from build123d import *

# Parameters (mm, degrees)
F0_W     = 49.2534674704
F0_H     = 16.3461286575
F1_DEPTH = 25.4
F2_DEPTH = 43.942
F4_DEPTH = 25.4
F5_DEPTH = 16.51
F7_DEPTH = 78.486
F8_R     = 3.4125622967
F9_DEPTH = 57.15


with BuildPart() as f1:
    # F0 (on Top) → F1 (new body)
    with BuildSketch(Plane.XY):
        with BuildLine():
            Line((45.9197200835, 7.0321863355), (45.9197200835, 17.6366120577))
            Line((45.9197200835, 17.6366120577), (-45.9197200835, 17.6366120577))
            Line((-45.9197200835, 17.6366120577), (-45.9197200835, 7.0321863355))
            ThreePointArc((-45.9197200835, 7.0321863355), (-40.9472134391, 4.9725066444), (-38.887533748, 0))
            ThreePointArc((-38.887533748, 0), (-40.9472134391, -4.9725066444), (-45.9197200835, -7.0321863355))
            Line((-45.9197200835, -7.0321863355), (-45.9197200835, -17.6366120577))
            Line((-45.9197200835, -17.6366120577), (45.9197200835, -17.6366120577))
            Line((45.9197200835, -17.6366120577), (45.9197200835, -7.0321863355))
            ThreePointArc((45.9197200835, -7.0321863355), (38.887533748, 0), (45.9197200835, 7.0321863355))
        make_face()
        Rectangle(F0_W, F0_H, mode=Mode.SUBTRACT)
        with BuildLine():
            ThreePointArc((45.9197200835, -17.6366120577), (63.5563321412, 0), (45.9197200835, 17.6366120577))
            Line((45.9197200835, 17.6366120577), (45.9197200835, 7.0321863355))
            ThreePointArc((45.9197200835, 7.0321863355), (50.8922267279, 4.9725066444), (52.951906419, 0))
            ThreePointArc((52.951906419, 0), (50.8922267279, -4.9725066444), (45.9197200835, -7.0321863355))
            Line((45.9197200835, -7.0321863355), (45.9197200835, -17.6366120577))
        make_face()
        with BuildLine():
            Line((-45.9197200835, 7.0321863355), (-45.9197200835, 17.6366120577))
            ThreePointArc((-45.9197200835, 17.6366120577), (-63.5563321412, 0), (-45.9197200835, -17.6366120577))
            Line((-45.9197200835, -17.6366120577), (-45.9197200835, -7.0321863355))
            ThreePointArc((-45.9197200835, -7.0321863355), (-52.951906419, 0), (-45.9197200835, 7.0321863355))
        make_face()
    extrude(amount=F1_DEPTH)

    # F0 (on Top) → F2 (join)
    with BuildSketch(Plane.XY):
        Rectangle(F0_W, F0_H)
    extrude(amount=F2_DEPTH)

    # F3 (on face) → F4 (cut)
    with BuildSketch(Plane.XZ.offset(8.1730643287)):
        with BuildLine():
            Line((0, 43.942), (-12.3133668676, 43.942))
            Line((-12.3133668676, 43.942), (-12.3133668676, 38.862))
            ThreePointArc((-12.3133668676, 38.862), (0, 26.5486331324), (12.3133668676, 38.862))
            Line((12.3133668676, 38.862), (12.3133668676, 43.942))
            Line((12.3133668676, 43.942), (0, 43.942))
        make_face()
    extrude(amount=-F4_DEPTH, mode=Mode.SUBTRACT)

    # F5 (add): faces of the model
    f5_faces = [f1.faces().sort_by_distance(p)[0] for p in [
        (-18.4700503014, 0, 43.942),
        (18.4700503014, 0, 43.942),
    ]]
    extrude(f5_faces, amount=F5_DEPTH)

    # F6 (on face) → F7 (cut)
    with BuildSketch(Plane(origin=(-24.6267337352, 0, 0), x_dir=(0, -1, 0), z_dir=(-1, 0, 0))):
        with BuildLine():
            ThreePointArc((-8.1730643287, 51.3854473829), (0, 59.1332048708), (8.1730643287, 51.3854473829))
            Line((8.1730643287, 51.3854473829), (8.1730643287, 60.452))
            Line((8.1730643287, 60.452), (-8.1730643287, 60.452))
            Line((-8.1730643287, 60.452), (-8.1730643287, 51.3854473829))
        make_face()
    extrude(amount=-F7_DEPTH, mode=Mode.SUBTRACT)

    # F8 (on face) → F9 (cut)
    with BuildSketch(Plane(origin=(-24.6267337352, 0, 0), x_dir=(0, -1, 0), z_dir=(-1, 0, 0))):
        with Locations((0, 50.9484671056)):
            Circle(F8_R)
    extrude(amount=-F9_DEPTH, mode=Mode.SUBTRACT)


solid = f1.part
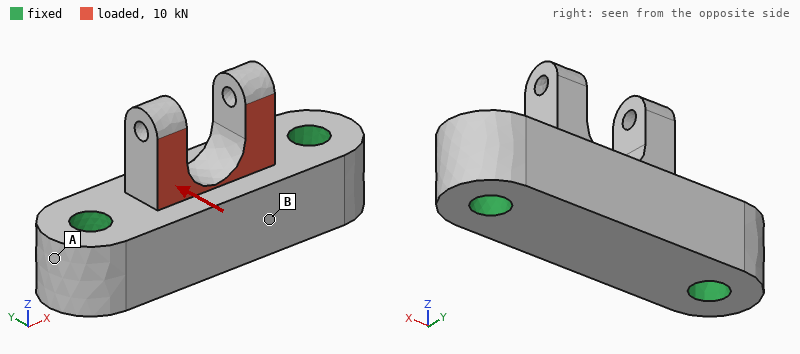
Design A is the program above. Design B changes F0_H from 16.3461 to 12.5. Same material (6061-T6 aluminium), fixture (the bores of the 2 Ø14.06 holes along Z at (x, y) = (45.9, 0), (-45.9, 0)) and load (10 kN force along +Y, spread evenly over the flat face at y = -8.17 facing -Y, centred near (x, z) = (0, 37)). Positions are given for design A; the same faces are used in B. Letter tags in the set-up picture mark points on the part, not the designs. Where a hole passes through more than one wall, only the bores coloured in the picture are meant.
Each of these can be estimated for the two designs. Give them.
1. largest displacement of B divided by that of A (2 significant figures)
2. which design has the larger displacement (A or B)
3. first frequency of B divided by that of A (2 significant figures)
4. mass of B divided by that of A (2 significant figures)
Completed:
1.9
B
0.93
0.97
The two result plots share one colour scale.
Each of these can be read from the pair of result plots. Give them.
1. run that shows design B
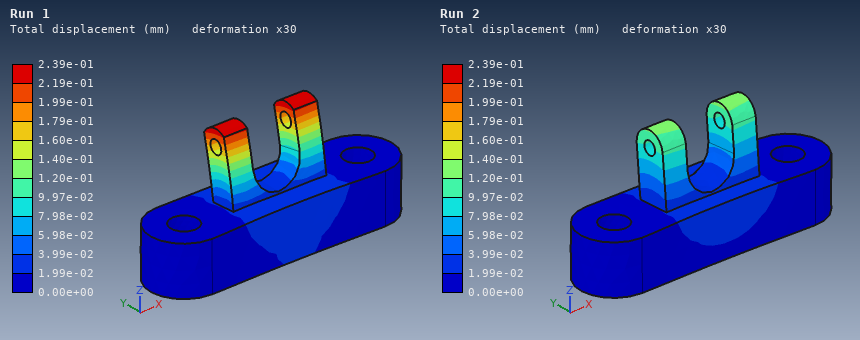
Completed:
Run 1
